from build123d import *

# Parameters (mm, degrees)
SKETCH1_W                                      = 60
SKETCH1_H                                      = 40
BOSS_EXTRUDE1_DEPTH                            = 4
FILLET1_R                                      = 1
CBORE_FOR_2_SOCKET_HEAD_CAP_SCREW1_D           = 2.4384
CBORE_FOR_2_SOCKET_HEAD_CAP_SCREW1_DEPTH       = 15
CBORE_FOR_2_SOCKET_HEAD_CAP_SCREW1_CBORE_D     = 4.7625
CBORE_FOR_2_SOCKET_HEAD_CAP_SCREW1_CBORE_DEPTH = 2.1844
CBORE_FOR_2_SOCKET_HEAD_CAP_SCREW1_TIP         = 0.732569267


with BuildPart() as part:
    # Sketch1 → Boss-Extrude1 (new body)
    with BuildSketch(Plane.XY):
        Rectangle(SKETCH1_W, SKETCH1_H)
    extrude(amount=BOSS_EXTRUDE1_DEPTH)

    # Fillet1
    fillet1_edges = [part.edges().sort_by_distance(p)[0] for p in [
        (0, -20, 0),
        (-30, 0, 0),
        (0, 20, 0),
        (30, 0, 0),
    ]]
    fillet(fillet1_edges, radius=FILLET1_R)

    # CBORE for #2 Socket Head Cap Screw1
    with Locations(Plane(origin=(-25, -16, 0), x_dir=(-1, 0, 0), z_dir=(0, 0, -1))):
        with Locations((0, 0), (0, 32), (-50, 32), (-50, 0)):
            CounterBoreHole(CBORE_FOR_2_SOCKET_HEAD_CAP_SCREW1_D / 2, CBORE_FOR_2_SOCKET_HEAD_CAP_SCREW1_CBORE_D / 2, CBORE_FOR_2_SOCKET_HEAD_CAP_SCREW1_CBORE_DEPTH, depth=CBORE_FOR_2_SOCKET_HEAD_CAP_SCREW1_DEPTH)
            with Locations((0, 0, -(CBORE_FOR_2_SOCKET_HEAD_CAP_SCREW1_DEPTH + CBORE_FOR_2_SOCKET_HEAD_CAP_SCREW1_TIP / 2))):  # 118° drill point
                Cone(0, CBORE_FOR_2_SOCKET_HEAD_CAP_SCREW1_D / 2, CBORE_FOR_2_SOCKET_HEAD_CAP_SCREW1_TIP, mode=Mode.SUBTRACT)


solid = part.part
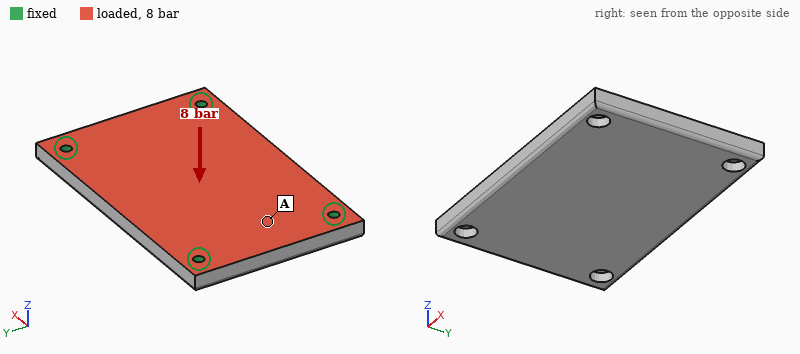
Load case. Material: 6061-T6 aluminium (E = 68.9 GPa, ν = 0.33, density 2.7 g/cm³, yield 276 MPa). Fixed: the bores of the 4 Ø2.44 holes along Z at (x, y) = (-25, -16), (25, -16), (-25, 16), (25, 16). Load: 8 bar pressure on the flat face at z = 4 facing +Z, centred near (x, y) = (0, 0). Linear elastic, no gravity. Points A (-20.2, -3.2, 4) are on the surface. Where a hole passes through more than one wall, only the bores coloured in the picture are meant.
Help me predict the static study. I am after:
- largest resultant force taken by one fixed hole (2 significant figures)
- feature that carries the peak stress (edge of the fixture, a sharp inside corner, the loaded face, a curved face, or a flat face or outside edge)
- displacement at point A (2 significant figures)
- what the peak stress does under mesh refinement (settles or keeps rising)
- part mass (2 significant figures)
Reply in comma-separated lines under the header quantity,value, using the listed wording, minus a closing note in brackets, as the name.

quantity,value
largest resultant force taken by one fixed hole,740 N
feature that carries the peak stress,edge of the fixture
displacement at point A,35 µm
what the peak stress does under mesh refinement,keeps rising
part mass,25 g
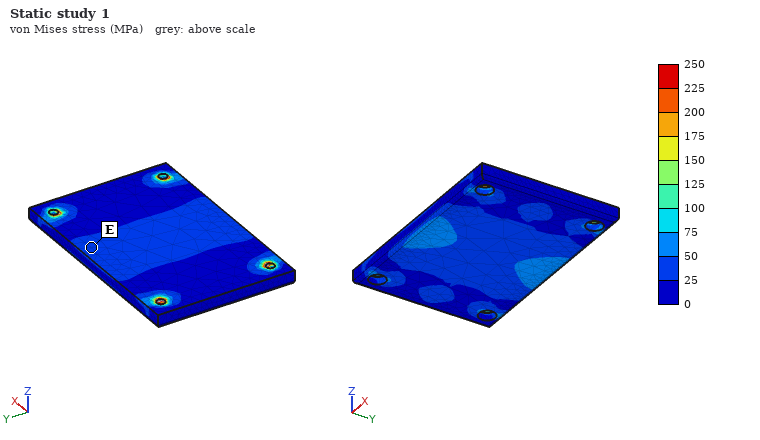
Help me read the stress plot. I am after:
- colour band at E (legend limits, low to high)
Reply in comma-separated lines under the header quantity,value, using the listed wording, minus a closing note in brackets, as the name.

quantity,value
colour band at E,25 to 50 MPa
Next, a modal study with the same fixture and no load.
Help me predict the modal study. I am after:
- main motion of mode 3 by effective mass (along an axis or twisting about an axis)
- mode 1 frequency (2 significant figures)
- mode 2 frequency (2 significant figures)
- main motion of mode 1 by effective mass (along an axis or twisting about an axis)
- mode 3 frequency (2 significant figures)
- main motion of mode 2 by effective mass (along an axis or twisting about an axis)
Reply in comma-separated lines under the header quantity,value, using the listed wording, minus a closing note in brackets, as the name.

quantity,value
main motion of mode 3 by effective mass,twisting about Y
mode 1 frequency,5400 Hz
mode 2 frequency,8700 Hz
main motion of mode 1 by effective mass,along Z
mode 3 frequency,13 kHz
main motion of mode 2 by effective mass,twisting about X
